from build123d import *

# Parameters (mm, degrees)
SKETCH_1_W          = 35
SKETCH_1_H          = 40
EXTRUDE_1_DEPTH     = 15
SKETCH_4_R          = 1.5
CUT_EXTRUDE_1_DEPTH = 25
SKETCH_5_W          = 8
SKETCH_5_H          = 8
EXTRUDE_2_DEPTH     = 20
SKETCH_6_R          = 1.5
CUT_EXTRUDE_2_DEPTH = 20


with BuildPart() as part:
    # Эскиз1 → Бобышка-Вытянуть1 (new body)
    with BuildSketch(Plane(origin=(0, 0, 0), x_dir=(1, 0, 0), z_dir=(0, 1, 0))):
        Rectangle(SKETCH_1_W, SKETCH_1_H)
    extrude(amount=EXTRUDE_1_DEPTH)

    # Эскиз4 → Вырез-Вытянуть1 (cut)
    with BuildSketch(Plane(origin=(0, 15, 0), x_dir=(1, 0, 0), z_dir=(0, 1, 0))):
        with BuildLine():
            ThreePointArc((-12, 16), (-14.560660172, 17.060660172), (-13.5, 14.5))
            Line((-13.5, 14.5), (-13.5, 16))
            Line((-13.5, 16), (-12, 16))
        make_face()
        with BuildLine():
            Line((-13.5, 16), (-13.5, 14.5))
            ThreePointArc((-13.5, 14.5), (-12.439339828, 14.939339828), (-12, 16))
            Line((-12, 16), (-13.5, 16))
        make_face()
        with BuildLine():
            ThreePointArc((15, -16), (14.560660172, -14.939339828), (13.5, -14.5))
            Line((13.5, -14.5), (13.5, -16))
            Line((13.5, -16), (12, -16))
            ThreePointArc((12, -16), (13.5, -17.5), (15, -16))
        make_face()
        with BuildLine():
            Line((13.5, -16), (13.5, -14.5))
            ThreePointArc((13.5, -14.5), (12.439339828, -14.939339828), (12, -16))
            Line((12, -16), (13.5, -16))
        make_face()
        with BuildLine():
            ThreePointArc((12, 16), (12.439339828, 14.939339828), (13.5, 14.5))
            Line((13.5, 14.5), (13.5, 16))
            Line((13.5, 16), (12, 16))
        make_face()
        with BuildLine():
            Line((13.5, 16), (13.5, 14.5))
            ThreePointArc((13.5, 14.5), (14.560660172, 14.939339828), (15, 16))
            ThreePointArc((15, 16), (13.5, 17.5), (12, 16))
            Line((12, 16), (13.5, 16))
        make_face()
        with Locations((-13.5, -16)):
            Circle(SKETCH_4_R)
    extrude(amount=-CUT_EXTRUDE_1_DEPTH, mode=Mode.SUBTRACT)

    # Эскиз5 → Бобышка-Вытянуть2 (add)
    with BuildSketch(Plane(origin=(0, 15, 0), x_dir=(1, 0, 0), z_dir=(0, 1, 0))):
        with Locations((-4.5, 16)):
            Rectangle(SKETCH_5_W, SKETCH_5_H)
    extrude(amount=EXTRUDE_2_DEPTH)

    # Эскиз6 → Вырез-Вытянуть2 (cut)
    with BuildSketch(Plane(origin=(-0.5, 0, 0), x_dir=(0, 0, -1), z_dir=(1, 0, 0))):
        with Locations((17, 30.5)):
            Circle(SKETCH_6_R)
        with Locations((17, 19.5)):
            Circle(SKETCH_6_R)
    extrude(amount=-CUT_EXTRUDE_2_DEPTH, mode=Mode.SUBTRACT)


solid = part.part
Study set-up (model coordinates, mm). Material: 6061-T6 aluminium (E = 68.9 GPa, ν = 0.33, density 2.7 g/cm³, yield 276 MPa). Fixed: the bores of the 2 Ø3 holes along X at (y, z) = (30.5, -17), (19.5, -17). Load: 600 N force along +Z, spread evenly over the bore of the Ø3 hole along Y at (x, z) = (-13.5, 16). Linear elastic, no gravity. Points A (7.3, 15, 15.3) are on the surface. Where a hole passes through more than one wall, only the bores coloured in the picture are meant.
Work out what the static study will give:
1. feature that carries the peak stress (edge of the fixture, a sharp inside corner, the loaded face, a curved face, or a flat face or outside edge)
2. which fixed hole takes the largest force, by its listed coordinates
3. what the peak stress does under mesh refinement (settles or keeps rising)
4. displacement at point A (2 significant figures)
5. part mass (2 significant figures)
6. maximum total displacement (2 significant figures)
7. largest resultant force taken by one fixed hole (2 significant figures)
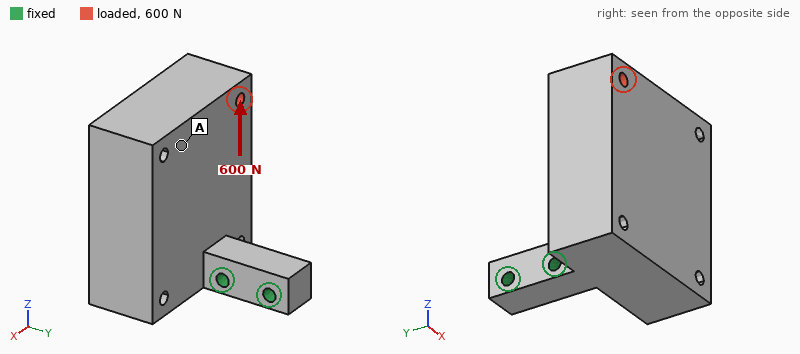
edge of the fixture
(19.5, -17)
keeps rising
0.091 mm
59 g
0.12 mm
890 N
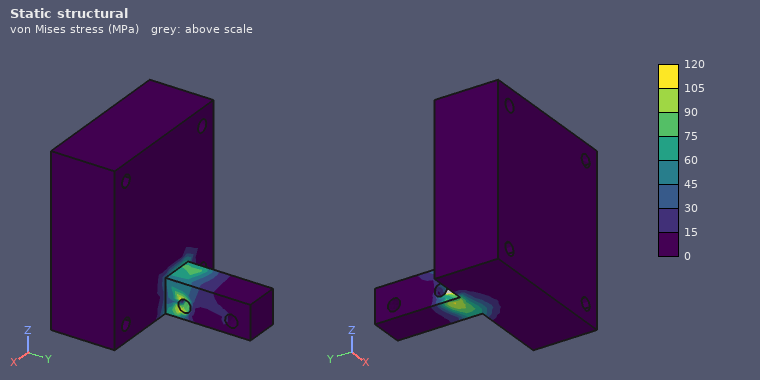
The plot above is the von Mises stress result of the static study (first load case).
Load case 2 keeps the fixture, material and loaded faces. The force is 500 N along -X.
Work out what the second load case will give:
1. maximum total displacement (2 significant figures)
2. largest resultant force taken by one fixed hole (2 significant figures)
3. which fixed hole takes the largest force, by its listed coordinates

0.27 mm
520 N
(19.5, -17)
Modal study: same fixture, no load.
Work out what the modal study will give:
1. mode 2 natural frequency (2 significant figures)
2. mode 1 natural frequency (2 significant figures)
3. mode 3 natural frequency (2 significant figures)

1600 Hz
1500 Hz
3200 Hz
